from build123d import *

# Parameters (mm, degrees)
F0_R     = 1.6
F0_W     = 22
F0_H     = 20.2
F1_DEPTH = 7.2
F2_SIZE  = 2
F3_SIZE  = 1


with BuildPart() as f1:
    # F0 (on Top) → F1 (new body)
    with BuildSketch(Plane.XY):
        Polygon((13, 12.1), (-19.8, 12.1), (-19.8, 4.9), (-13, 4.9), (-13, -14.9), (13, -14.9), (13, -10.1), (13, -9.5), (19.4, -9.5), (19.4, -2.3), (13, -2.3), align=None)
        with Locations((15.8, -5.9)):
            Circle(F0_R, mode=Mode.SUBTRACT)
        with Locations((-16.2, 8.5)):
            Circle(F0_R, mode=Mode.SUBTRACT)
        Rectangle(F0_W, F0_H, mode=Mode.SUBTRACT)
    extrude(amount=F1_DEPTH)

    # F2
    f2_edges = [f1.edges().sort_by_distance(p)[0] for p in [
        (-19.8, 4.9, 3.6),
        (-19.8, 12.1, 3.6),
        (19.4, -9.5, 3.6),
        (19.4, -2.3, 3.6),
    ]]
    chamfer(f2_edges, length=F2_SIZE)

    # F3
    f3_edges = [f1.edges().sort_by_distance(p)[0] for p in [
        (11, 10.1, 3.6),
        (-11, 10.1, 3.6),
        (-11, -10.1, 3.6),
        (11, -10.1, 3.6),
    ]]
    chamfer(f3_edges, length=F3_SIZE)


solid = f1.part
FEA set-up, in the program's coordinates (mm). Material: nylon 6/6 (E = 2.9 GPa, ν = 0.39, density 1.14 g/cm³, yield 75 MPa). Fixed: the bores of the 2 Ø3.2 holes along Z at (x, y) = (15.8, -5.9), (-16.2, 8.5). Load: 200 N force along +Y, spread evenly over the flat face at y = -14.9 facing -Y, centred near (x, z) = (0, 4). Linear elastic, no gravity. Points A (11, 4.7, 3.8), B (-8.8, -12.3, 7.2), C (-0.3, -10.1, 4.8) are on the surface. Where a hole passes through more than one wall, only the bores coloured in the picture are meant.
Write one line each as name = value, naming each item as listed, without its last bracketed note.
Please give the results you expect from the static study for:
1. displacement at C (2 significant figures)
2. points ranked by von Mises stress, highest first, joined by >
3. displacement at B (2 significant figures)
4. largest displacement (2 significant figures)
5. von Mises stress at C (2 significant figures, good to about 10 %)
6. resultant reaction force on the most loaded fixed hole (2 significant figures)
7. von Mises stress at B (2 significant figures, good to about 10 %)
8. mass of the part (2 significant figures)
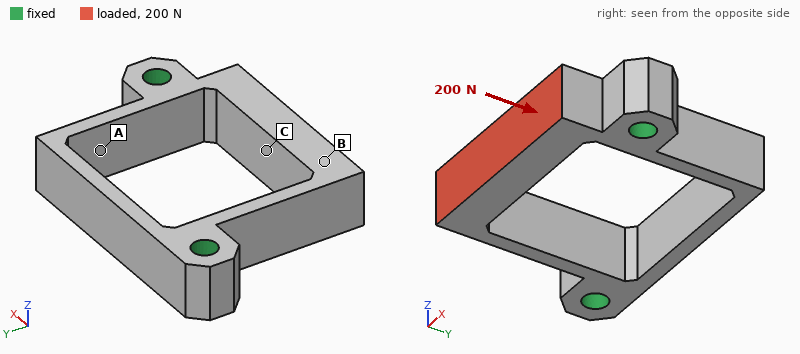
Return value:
displacement at C = 0.18 mm
points ranked by von Mises stress, highest first, joined by > = C > B > A
displacement at B = 0.12 mm
largest displacement = 0.18 mm
von Mises stress at C = 15 MPa
resultant reaction force on the most loaded fixed hole = 100 N
von Mises stress at B = 6.7 MPa
mass of the part = 2.7 g
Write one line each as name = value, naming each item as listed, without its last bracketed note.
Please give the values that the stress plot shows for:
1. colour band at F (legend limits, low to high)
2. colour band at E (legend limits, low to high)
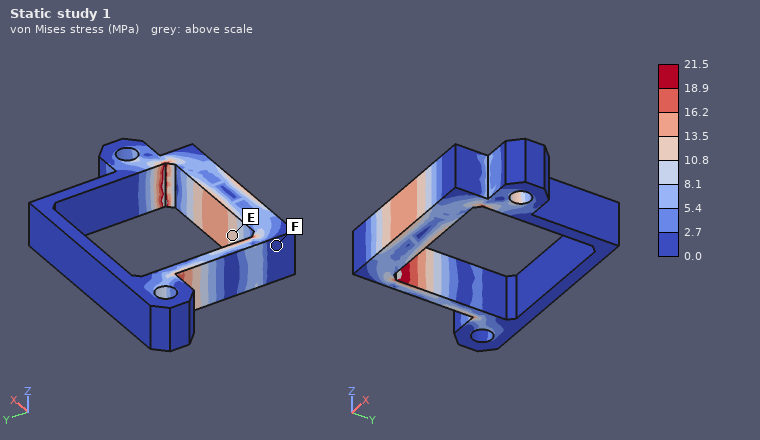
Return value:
colour band at F = 0.0 to 2.7 MPa
colour band at E = 10.8 to 13.5 MPa
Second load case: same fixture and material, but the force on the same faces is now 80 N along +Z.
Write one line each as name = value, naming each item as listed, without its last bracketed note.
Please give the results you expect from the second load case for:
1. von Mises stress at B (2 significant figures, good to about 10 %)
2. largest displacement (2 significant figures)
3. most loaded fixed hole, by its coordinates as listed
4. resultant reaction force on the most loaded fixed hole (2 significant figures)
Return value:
von Mises stress at B = 3.2 MPa
largest displacement = 0.48 mm
most loaded fixed hole, by its coordinates as listed = (15.8, -5.9)
resultant reaction force on the most loaded fixed hole = 56 N
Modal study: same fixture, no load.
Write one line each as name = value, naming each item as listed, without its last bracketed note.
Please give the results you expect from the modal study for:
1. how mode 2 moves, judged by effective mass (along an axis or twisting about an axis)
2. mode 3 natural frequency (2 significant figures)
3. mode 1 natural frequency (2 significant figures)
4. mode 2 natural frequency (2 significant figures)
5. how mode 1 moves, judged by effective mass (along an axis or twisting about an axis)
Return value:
how mode 2 moves, judged by effective mass = along Z
mode 3 natural frequency = 4700 Hz
mode 1 natural frequency = 2600 Hz
mode 2 natural frequency = 4200 Hz
how mode 1 moves, judged by effective mass = along Z
